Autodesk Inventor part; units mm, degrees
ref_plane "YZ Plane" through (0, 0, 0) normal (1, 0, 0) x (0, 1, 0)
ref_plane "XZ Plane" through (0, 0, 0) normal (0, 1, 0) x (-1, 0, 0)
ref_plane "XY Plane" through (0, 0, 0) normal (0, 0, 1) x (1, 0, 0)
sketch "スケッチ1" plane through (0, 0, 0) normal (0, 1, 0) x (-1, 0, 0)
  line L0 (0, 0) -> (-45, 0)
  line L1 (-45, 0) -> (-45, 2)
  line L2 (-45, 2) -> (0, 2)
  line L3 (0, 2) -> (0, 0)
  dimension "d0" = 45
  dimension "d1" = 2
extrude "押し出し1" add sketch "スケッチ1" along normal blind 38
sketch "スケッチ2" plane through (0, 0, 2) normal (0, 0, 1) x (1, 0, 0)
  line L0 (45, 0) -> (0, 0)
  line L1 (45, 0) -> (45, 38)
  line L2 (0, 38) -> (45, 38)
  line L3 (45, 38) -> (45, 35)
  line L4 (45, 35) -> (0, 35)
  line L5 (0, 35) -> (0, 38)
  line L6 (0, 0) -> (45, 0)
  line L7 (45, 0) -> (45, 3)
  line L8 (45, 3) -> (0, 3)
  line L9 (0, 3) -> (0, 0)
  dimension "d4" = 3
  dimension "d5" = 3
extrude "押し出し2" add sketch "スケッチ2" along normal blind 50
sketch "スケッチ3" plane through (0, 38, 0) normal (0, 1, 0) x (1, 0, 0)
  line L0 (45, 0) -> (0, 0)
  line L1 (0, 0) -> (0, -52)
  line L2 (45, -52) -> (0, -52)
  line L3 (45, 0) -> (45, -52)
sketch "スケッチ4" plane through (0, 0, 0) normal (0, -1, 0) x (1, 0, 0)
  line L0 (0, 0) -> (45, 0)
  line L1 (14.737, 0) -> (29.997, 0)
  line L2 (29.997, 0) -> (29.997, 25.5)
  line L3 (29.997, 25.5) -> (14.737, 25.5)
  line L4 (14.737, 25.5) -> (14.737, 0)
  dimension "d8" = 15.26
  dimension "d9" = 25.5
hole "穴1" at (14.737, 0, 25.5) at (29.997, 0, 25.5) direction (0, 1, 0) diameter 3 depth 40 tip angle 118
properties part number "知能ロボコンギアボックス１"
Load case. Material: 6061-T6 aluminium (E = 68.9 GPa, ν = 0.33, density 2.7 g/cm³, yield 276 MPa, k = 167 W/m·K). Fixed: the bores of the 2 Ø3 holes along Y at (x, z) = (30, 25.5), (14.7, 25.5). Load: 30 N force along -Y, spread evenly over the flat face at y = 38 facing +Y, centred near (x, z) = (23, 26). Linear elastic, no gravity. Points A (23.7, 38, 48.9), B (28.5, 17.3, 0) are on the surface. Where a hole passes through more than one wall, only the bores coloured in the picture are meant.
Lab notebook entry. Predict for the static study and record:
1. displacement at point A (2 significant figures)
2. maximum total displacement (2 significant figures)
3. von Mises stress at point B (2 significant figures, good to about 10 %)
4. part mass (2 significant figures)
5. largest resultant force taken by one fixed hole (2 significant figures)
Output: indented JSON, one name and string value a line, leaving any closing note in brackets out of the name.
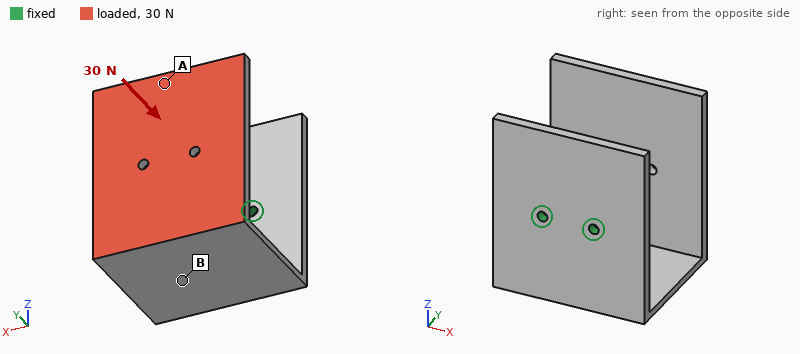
{
  "displacement at point A": "0.69 mm",
  "maximum total displacement": "0.73 mm",
  "von Mises stress at point B": "22 MPa",
  "part mass": "45 g",
  "largest resultant force taken by one fixed hole": "15 N"
}
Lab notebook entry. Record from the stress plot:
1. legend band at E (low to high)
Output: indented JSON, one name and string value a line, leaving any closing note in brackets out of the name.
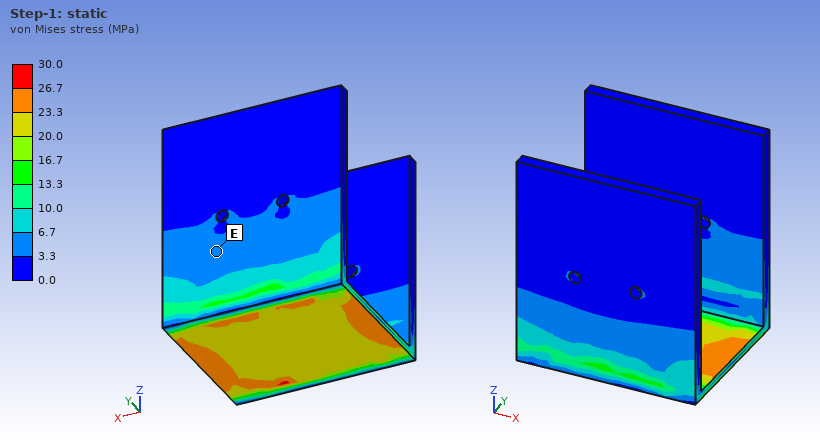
{
  "legend band at E": "3.3 to 6.7 MPa"
}
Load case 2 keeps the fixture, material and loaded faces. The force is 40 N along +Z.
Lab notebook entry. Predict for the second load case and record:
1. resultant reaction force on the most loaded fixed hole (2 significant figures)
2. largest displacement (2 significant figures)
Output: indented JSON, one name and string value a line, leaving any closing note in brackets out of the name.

{
  "resultant reaction force on the most loaded fixed hole": "21 N",
  "largest displacement": "0.89 mm"
}
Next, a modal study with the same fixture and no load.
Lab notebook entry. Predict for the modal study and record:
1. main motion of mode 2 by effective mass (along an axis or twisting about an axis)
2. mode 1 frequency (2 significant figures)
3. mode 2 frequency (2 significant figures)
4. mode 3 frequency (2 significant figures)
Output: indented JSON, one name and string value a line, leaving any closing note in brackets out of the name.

{
  "main motion of mode 2 by effective mass": "along X",
  "mode 1 frequency": "240 Hz",
  "mode 2 frequency": "390 Hz",
  "mode 3 frequency": "660 Hz"
}
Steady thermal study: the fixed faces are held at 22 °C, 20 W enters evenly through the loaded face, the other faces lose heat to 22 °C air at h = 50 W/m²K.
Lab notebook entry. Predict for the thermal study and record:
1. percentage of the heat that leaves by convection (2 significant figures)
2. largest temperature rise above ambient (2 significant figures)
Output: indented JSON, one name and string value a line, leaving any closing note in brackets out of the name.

{
  "percentage of the heat that leaves by convection": "56 %",
  "largest temperature rise above ambient": "51 K"
}
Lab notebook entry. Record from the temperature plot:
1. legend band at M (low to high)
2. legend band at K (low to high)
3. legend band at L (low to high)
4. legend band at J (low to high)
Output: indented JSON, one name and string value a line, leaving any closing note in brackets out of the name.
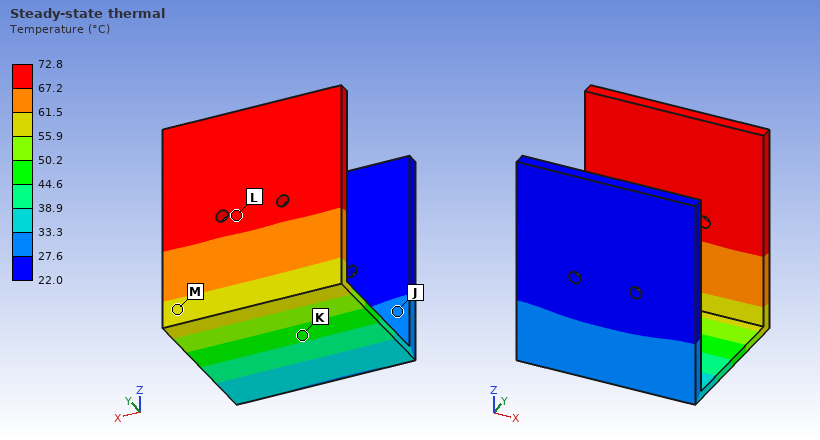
{
  "legend band at M": "55.9 to 61.5 °C",
  "legend band at K": "44.6 to 50.2 °C",
  "legend band at L": "67.2 to 72.8 °C",
  "legend band at J": "27.6 to 33.3 °C"
}
